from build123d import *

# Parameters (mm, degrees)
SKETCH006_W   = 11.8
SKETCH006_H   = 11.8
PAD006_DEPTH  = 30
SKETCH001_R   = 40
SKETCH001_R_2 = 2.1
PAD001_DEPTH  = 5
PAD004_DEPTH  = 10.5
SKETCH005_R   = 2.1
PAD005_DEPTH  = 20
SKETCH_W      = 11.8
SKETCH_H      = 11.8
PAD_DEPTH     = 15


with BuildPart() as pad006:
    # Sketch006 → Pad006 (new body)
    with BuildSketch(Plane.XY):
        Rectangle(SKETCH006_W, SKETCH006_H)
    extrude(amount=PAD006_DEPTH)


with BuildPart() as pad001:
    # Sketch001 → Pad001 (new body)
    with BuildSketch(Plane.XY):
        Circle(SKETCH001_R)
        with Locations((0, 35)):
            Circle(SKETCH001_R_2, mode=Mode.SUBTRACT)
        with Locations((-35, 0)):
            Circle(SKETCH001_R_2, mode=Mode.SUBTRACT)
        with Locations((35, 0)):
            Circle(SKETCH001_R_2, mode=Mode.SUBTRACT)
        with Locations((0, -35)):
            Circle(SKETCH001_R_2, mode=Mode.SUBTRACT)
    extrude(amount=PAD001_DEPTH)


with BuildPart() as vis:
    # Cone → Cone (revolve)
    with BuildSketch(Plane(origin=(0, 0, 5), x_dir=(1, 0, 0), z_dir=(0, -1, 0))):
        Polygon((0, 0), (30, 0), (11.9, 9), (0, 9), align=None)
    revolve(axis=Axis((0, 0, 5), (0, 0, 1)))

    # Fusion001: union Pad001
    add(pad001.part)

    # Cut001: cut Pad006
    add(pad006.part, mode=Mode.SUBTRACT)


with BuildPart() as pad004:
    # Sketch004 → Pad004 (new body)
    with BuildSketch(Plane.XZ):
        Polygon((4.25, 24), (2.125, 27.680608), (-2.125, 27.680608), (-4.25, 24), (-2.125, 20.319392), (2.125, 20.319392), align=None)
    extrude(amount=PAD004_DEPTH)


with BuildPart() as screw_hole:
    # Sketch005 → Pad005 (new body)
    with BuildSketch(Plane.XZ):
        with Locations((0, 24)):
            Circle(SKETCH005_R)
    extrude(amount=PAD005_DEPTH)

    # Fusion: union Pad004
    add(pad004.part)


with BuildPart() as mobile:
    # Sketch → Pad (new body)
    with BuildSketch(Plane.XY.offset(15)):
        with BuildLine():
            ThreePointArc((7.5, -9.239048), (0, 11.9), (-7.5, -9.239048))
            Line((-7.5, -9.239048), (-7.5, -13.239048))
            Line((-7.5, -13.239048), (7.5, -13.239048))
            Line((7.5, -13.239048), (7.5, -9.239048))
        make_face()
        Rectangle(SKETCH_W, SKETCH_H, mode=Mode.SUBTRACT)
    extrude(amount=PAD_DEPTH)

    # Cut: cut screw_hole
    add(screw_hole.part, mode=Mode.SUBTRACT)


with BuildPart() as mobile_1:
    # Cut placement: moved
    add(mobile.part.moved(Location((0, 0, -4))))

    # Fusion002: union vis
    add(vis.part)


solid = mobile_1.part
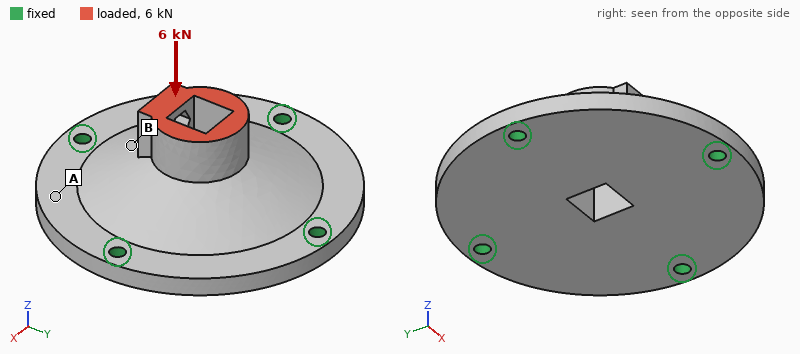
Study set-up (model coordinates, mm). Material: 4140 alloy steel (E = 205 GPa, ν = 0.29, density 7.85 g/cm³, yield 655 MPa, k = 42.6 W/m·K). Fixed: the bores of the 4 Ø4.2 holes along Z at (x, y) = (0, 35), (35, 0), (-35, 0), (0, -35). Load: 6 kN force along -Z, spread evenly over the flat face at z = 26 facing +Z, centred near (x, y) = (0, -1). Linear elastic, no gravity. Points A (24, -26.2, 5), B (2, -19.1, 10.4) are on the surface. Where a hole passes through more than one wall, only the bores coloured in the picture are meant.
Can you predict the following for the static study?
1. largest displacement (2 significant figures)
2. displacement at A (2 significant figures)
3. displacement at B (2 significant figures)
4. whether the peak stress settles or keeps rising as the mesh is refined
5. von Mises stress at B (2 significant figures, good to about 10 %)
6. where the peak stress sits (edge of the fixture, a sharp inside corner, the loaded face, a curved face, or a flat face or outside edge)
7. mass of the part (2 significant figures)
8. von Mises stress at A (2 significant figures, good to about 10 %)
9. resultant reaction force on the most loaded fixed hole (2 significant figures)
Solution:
14 µm
6.6 µm
9.6 µm
keeps rising
36 MPa
edge of the fixture
310 g
14 MPa
2.1 kN
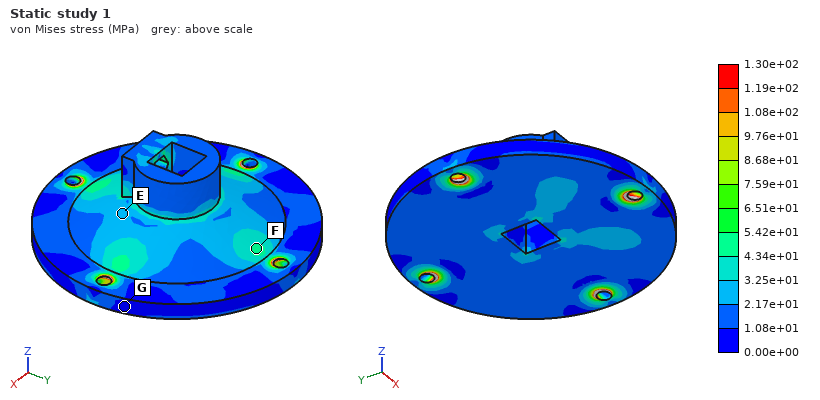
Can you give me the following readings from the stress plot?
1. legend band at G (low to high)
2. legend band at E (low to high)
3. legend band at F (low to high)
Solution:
0.00e+00 to 1.08e+01 MPa
2.17e+01 to 3.25e+01 MPa
4.34e+01 to 5.42e+01 MPa
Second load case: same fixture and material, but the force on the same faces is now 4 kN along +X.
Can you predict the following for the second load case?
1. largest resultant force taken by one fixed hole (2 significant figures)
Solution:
2.2 kN
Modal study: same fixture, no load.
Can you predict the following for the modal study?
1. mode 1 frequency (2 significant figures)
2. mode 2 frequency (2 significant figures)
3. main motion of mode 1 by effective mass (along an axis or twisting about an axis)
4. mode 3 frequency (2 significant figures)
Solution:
8200 Hz
10 kHz
along Z
10 kHz
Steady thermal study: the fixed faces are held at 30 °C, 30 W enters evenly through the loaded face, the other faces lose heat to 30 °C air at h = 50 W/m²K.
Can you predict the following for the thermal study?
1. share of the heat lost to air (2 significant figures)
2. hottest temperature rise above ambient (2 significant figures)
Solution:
32 %
59 K
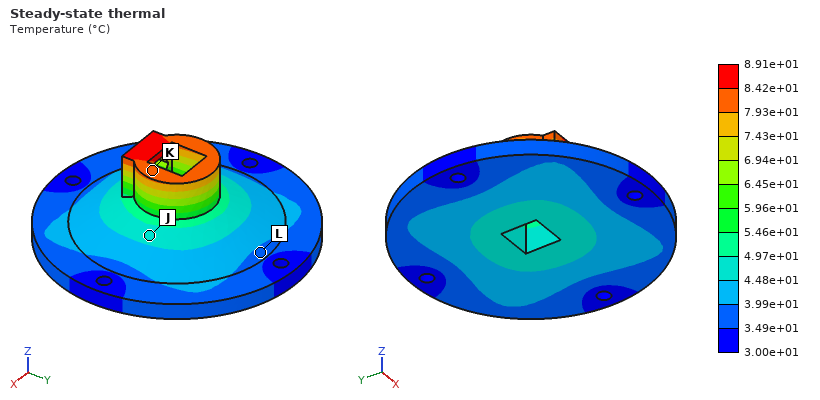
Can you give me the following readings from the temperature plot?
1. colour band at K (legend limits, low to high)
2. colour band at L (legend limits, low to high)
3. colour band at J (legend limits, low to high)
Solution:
7.93e+01 to 8.42e+01 °C
3.49e+01 to 3.99e+01 °C
4.48e+01 to 4.97e+01 °C
